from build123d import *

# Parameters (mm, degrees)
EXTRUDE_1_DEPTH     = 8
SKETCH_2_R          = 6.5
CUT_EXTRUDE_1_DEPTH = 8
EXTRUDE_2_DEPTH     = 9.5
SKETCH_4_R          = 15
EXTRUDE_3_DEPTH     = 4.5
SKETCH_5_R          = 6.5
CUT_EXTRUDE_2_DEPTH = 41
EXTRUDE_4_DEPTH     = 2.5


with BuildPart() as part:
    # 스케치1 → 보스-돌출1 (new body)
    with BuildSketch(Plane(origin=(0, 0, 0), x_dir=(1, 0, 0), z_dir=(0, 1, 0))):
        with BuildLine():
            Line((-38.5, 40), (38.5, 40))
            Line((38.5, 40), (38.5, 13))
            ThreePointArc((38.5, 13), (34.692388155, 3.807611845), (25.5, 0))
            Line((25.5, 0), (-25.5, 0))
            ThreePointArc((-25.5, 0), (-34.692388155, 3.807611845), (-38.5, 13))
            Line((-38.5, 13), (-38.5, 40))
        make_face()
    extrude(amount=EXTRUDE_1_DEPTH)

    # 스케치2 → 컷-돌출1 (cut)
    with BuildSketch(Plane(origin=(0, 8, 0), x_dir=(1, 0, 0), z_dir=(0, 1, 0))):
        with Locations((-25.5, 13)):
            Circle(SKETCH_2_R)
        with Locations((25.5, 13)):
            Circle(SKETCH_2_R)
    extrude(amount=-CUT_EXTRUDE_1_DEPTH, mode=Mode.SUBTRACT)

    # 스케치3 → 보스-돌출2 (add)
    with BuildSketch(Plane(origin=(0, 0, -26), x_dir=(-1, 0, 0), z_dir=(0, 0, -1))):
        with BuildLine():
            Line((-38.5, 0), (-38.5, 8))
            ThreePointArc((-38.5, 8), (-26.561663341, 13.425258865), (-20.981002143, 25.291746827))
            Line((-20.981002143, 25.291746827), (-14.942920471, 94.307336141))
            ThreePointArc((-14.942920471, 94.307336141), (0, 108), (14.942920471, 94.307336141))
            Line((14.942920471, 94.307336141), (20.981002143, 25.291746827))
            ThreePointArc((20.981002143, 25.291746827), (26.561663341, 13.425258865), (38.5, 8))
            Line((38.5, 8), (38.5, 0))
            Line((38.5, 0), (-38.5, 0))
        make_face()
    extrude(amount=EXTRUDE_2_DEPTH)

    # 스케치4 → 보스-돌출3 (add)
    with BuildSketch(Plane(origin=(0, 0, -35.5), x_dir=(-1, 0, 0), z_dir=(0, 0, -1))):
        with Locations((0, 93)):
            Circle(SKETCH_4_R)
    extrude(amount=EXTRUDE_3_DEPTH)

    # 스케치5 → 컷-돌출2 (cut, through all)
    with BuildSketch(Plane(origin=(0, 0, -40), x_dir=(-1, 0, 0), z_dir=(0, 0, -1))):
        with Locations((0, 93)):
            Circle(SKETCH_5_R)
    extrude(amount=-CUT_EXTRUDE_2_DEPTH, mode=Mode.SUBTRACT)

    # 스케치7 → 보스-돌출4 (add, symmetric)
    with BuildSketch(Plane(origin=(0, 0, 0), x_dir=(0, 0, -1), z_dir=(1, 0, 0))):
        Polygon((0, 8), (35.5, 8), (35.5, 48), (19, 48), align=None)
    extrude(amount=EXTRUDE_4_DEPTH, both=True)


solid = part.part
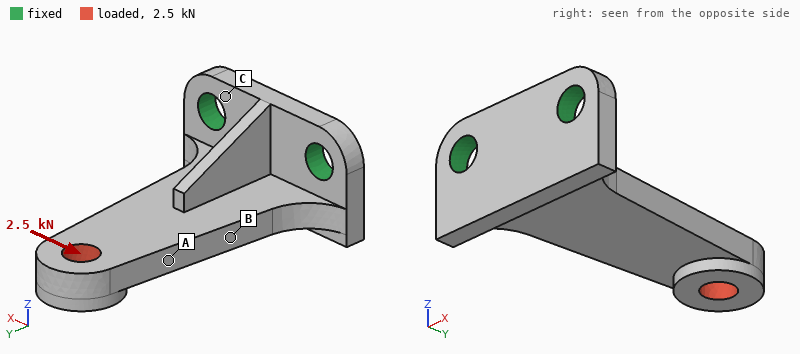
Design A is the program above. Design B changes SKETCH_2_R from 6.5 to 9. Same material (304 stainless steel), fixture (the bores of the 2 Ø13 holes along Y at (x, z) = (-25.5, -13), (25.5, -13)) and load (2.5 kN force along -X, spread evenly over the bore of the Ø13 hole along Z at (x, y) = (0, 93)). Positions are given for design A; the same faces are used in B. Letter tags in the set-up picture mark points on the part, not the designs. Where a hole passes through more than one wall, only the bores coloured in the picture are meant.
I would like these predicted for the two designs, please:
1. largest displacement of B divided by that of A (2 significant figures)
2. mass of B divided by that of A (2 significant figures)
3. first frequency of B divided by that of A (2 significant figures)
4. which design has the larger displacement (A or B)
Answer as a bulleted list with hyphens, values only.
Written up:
- 0.86
- 0.97
- 1.1
- A
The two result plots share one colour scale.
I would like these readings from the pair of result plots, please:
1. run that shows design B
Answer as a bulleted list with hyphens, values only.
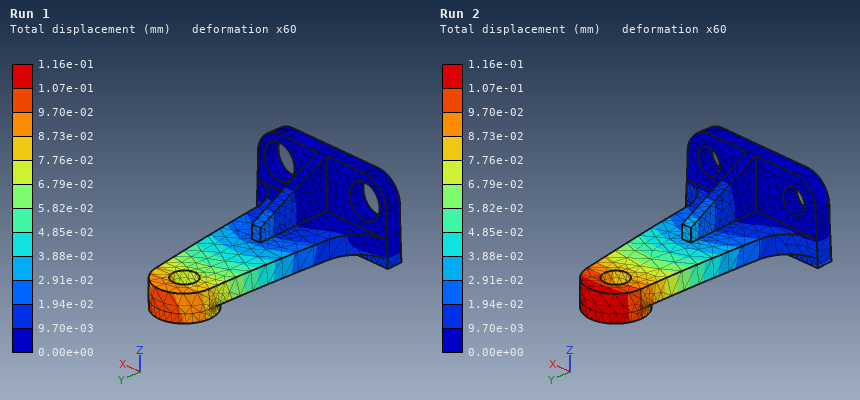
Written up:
- Run 1
